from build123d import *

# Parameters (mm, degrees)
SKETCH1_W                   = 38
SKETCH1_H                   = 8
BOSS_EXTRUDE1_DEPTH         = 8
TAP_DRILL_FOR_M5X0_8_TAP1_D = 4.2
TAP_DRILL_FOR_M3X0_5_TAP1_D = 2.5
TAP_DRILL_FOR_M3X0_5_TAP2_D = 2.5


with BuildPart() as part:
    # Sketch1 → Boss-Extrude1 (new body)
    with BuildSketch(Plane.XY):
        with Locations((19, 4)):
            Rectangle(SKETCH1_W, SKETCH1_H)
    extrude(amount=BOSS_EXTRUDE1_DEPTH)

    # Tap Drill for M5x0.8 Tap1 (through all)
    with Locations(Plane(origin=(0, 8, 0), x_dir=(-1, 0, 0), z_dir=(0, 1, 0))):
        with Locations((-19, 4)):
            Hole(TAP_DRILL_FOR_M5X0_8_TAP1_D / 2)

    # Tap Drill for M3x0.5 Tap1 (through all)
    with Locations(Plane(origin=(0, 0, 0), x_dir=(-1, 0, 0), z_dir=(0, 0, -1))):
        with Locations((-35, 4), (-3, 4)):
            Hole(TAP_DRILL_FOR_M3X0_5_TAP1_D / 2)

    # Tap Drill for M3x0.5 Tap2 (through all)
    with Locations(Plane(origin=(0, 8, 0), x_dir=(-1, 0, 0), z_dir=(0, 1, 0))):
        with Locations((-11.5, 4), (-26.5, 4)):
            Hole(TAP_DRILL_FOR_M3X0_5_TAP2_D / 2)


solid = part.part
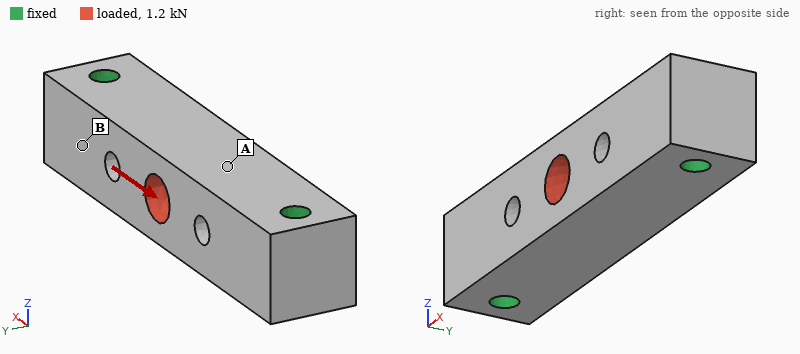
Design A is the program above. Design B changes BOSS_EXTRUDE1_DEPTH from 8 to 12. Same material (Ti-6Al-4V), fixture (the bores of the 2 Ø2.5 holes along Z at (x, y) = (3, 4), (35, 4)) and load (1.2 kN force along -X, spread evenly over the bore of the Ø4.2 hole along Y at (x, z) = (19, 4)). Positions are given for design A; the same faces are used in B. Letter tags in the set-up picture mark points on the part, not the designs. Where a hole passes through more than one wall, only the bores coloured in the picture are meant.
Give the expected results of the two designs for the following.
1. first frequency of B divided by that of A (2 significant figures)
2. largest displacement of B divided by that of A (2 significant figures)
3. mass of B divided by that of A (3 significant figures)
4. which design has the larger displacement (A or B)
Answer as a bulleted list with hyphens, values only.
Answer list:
- 1.0
- 0.87
- 1.54
- A
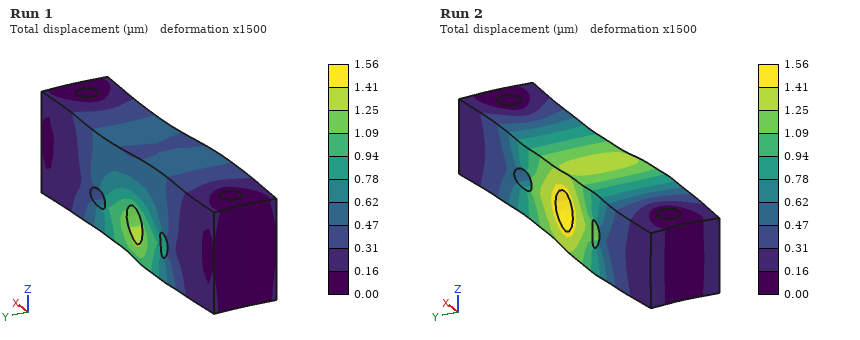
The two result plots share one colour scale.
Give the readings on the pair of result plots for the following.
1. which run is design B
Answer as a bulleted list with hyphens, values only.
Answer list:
- Run 1
